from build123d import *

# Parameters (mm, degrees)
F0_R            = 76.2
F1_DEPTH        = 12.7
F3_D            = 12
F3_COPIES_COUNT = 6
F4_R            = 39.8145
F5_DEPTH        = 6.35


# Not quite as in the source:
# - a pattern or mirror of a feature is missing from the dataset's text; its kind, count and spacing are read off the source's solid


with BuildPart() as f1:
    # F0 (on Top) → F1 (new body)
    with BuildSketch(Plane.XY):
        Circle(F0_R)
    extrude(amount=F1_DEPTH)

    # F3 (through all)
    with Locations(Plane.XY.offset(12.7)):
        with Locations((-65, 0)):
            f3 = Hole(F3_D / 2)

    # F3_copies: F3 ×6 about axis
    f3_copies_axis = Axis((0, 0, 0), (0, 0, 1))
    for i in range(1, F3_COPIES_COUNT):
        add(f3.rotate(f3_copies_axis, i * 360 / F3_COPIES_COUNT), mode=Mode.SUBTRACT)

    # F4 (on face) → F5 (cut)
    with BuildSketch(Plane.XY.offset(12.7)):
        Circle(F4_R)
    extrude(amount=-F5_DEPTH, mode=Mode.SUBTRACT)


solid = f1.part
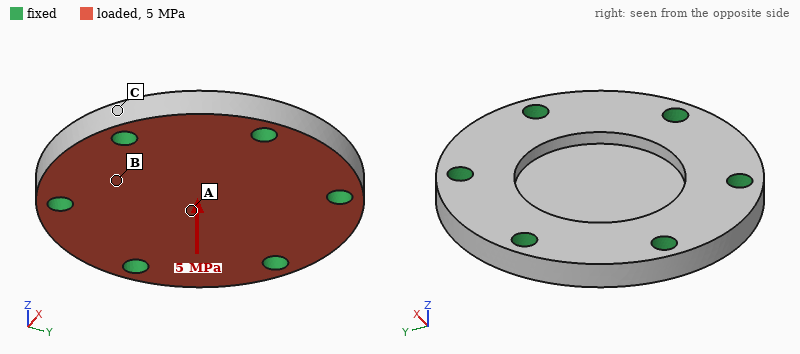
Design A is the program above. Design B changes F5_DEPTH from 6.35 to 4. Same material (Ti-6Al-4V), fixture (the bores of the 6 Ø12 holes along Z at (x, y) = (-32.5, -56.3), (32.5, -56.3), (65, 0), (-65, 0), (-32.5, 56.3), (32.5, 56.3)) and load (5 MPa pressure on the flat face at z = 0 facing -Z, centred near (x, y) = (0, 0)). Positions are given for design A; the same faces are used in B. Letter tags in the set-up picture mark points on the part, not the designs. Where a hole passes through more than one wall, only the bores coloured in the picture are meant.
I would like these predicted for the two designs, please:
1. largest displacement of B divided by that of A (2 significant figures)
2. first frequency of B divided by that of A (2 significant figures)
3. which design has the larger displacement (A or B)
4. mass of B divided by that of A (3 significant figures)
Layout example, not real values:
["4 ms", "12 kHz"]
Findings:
["0.67", "1.0", "A", "1.06"]
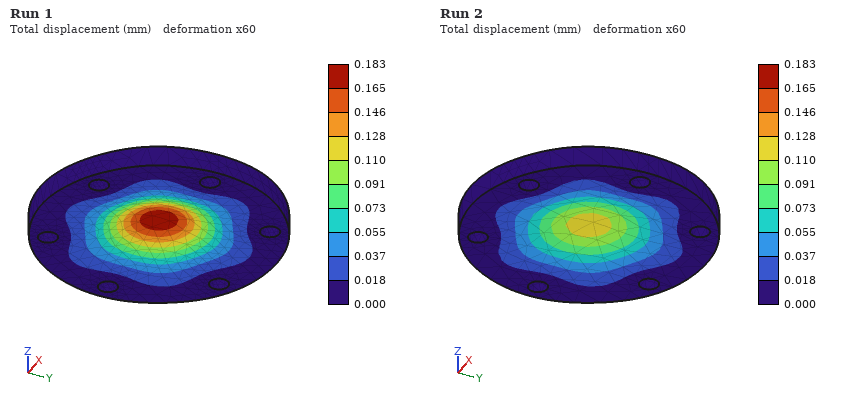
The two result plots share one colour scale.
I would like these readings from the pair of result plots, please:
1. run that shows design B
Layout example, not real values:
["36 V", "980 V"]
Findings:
["Run 2"]
